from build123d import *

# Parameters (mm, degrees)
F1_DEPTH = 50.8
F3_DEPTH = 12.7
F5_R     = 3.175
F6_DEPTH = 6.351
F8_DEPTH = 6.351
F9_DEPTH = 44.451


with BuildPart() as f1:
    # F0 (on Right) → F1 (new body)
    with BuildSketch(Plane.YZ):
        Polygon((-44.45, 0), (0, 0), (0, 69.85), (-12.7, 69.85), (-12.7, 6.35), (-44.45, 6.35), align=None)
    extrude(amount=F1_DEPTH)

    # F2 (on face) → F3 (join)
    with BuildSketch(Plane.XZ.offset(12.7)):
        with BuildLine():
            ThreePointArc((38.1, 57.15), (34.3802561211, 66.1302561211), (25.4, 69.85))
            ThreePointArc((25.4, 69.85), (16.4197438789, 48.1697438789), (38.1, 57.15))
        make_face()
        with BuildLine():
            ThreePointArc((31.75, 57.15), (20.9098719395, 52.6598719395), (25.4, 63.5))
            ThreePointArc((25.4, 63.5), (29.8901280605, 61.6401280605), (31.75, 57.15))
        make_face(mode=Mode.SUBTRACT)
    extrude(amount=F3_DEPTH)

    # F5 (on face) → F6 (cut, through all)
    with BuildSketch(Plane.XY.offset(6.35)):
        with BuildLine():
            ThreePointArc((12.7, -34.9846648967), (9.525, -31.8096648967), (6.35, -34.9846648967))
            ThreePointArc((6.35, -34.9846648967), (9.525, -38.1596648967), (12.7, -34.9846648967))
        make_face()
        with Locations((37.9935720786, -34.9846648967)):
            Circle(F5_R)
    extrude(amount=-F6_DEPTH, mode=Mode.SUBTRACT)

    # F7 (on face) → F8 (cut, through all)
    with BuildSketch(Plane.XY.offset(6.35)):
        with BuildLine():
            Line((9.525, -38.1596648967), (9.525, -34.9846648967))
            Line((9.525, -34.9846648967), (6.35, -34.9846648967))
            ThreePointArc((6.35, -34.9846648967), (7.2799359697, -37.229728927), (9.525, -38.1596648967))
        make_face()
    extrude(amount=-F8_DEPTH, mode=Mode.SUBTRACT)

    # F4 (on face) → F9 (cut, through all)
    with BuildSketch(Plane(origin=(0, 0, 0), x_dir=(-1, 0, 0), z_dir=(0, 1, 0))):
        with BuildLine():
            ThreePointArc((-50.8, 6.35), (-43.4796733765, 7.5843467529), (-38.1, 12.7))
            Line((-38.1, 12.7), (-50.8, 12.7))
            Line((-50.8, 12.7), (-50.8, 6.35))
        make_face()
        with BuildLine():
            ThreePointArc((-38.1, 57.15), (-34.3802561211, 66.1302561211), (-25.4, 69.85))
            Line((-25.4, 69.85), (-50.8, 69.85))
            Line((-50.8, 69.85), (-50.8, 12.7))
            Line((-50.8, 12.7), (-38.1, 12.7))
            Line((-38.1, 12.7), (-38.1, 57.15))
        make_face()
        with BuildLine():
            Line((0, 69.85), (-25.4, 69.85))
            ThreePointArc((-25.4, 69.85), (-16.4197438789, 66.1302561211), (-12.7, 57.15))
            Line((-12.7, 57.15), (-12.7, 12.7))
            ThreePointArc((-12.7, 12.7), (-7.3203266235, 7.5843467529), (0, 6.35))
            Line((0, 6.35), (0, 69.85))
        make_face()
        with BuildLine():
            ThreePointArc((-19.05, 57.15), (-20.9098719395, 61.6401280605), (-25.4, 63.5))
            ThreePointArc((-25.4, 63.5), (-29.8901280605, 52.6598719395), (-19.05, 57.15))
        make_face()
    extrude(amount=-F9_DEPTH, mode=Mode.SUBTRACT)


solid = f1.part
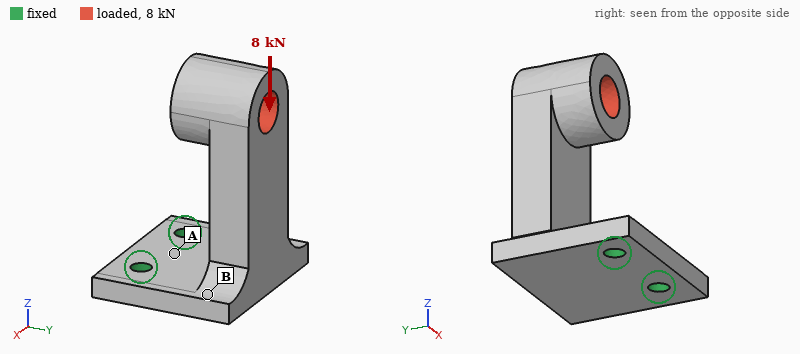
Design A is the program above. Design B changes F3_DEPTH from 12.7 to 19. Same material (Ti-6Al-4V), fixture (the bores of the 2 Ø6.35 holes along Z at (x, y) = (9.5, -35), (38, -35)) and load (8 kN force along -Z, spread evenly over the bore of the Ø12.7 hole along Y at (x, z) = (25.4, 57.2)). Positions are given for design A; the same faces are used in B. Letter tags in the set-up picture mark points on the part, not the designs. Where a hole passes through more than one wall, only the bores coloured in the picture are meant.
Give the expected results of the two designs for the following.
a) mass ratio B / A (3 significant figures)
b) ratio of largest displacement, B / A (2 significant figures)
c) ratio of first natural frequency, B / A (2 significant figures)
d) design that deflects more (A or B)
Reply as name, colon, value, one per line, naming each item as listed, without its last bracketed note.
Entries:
mass ratio B / A: 1.06
ratio of largest displacement, B / A: 0.51
ratio of first natural frequency, B / A: 0.92
design that deflects more: A
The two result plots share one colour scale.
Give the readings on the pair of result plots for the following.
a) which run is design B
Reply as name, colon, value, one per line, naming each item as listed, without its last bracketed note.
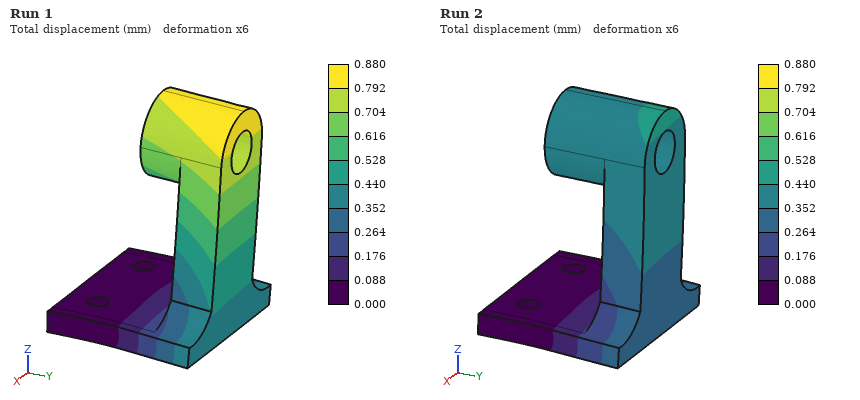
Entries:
which run is design B: Run 2
